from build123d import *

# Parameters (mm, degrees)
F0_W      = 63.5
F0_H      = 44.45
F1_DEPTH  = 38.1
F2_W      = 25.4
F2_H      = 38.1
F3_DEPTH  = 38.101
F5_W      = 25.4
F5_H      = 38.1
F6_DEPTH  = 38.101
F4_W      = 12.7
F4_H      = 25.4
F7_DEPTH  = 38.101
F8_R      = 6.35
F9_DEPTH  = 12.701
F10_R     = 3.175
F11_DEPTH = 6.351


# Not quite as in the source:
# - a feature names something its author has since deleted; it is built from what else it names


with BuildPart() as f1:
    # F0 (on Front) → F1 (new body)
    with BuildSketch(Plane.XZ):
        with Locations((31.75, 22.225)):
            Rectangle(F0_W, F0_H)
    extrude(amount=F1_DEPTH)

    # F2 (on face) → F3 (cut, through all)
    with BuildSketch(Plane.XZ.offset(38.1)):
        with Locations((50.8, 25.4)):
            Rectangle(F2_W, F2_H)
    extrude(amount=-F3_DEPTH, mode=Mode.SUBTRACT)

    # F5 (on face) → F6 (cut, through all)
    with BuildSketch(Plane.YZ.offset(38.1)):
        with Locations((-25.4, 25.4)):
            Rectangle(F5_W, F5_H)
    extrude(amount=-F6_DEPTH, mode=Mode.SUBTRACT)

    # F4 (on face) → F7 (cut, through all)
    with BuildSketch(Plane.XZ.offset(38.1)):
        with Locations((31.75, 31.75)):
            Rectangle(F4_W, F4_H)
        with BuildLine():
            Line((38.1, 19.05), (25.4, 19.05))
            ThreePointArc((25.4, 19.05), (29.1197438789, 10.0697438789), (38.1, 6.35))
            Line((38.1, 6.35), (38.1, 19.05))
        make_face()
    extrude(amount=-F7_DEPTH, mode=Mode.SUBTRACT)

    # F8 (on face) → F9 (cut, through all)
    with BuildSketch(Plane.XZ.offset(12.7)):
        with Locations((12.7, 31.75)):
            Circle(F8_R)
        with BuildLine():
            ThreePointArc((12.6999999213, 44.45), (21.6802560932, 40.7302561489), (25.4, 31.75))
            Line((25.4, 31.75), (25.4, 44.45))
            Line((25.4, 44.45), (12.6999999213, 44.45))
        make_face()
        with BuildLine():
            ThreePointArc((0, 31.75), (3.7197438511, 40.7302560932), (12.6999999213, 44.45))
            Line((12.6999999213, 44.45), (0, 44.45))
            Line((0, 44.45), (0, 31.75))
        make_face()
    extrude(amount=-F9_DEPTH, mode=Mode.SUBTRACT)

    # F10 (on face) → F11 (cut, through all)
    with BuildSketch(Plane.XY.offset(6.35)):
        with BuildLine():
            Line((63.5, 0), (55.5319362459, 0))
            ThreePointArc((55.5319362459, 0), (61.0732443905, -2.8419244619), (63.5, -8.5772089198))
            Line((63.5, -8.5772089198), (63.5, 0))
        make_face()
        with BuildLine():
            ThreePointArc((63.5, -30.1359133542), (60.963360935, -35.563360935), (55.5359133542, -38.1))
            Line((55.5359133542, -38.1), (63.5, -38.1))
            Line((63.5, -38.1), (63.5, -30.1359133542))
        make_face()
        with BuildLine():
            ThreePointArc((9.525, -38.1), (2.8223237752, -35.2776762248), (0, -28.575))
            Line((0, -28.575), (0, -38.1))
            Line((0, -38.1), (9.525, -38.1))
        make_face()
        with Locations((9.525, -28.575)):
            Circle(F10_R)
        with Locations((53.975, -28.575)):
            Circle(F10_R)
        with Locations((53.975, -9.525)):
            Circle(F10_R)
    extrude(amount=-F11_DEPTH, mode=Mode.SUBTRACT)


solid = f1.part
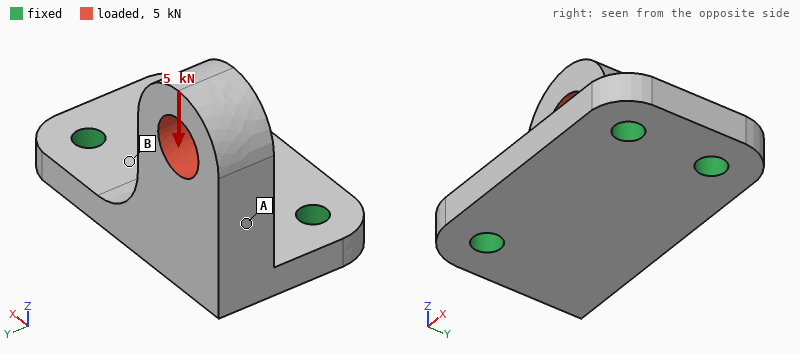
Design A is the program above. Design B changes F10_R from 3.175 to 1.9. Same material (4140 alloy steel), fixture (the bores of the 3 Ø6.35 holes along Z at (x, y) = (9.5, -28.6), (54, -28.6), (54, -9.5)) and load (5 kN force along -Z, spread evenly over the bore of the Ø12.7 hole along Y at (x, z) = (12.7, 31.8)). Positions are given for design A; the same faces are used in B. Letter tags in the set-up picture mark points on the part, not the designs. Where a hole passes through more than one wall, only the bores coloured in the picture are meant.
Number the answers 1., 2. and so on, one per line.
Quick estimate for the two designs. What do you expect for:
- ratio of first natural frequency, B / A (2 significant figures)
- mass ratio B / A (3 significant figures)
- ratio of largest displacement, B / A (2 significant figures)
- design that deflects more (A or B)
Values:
1. 0.93
2. 1.02
3. 1.2
4. B
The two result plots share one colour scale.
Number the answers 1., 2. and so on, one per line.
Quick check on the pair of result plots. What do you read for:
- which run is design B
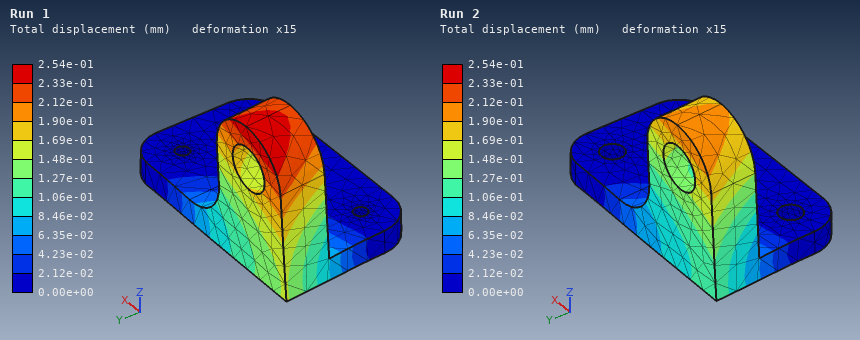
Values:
1. Run 1
